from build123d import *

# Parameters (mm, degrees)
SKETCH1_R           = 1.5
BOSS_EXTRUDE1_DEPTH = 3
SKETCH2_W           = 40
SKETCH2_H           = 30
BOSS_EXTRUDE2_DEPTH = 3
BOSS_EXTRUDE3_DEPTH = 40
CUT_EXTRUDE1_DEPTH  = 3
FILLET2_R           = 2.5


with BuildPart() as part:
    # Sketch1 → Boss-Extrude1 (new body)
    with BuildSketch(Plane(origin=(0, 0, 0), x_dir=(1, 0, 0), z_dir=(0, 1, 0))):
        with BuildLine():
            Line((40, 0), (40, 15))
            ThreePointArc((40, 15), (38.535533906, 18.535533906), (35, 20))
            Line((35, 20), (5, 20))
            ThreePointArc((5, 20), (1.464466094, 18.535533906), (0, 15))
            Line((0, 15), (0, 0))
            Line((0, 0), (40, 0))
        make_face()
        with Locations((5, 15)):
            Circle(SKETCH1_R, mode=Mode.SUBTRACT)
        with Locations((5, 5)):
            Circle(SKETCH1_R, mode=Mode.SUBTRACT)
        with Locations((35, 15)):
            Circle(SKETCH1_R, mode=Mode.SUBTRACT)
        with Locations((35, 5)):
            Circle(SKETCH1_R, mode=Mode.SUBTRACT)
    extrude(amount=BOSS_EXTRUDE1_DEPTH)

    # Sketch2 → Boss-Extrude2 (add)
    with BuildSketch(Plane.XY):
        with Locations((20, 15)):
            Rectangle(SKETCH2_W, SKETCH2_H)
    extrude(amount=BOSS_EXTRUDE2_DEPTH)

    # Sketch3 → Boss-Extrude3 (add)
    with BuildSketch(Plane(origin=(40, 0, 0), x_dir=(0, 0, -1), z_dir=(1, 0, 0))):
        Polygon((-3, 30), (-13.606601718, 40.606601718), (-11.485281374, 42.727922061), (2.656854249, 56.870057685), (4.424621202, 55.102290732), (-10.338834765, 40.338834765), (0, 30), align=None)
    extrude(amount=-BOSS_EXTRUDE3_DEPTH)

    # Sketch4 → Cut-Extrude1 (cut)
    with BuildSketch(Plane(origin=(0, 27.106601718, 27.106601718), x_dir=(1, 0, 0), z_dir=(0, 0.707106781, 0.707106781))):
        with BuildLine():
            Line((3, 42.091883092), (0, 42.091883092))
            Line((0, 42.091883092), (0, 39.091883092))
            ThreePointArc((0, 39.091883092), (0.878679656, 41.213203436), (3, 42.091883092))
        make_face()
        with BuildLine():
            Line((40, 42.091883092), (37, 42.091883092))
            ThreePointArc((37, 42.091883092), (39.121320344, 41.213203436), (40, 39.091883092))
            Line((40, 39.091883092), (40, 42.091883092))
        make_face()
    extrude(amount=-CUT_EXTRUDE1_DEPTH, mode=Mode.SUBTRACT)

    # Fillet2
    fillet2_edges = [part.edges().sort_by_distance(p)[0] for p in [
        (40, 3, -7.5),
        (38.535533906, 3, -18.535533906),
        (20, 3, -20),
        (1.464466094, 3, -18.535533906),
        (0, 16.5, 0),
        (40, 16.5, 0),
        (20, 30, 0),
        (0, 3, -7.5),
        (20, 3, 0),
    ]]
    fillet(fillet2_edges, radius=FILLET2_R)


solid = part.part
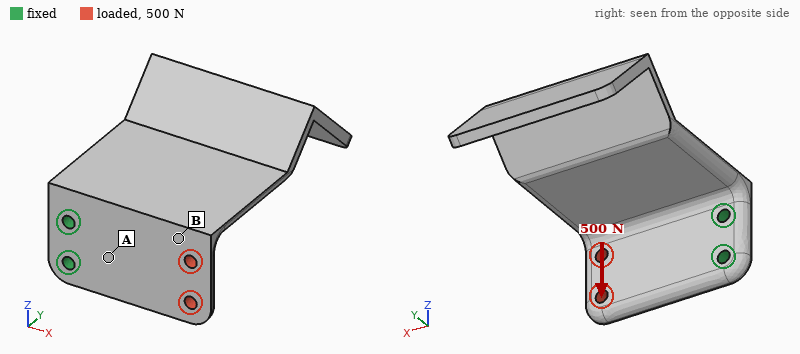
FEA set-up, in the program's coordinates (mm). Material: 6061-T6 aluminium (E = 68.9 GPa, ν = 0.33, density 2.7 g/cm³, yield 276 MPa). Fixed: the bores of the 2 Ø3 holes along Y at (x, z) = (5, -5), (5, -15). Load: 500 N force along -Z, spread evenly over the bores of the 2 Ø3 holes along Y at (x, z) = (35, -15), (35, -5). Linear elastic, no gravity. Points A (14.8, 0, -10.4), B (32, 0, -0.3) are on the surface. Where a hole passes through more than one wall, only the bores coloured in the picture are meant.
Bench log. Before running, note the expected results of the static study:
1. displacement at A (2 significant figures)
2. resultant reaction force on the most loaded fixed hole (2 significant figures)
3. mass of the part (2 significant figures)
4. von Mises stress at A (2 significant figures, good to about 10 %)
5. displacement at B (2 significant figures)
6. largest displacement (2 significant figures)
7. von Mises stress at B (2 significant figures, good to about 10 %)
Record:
10 µm
1.2 kN
25 g
26 MPa
40 µm
54 µm
12 MPa
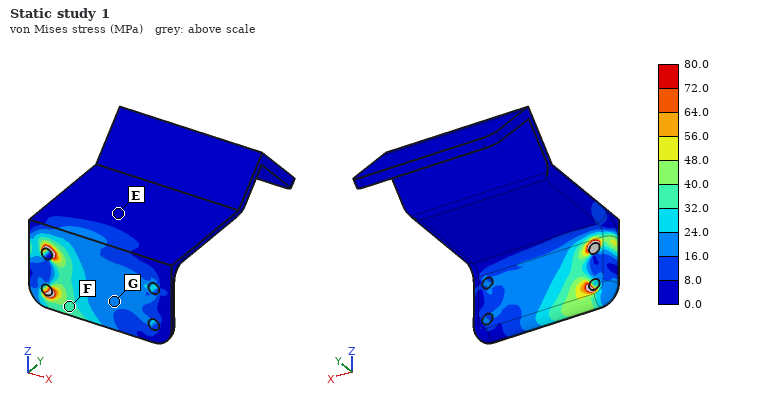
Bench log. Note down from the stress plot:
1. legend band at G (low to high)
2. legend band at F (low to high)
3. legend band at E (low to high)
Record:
16.0 to 24.0 MPa
32.0 to 40.0 MPa
0.0 to 8.0 MPa
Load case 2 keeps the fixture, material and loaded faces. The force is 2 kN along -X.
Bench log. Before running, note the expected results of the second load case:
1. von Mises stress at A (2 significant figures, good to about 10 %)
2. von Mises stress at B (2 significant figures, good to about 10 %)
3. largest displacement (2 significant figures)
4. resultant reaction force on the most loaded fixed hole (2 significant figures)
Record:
34 MPa
16 MPa
21 µm
1.0 kN
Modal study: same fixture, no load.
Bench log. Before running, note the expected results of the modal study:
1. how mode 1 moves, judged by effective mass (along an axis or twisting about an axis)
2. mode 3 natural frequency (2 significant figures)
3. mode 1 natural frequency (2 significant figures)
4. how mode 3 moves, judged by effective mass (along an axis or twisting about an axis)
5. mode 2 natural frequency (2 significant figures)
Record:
along Z
1900 Hz
560 Hz
twisting about Y
880 Hz
